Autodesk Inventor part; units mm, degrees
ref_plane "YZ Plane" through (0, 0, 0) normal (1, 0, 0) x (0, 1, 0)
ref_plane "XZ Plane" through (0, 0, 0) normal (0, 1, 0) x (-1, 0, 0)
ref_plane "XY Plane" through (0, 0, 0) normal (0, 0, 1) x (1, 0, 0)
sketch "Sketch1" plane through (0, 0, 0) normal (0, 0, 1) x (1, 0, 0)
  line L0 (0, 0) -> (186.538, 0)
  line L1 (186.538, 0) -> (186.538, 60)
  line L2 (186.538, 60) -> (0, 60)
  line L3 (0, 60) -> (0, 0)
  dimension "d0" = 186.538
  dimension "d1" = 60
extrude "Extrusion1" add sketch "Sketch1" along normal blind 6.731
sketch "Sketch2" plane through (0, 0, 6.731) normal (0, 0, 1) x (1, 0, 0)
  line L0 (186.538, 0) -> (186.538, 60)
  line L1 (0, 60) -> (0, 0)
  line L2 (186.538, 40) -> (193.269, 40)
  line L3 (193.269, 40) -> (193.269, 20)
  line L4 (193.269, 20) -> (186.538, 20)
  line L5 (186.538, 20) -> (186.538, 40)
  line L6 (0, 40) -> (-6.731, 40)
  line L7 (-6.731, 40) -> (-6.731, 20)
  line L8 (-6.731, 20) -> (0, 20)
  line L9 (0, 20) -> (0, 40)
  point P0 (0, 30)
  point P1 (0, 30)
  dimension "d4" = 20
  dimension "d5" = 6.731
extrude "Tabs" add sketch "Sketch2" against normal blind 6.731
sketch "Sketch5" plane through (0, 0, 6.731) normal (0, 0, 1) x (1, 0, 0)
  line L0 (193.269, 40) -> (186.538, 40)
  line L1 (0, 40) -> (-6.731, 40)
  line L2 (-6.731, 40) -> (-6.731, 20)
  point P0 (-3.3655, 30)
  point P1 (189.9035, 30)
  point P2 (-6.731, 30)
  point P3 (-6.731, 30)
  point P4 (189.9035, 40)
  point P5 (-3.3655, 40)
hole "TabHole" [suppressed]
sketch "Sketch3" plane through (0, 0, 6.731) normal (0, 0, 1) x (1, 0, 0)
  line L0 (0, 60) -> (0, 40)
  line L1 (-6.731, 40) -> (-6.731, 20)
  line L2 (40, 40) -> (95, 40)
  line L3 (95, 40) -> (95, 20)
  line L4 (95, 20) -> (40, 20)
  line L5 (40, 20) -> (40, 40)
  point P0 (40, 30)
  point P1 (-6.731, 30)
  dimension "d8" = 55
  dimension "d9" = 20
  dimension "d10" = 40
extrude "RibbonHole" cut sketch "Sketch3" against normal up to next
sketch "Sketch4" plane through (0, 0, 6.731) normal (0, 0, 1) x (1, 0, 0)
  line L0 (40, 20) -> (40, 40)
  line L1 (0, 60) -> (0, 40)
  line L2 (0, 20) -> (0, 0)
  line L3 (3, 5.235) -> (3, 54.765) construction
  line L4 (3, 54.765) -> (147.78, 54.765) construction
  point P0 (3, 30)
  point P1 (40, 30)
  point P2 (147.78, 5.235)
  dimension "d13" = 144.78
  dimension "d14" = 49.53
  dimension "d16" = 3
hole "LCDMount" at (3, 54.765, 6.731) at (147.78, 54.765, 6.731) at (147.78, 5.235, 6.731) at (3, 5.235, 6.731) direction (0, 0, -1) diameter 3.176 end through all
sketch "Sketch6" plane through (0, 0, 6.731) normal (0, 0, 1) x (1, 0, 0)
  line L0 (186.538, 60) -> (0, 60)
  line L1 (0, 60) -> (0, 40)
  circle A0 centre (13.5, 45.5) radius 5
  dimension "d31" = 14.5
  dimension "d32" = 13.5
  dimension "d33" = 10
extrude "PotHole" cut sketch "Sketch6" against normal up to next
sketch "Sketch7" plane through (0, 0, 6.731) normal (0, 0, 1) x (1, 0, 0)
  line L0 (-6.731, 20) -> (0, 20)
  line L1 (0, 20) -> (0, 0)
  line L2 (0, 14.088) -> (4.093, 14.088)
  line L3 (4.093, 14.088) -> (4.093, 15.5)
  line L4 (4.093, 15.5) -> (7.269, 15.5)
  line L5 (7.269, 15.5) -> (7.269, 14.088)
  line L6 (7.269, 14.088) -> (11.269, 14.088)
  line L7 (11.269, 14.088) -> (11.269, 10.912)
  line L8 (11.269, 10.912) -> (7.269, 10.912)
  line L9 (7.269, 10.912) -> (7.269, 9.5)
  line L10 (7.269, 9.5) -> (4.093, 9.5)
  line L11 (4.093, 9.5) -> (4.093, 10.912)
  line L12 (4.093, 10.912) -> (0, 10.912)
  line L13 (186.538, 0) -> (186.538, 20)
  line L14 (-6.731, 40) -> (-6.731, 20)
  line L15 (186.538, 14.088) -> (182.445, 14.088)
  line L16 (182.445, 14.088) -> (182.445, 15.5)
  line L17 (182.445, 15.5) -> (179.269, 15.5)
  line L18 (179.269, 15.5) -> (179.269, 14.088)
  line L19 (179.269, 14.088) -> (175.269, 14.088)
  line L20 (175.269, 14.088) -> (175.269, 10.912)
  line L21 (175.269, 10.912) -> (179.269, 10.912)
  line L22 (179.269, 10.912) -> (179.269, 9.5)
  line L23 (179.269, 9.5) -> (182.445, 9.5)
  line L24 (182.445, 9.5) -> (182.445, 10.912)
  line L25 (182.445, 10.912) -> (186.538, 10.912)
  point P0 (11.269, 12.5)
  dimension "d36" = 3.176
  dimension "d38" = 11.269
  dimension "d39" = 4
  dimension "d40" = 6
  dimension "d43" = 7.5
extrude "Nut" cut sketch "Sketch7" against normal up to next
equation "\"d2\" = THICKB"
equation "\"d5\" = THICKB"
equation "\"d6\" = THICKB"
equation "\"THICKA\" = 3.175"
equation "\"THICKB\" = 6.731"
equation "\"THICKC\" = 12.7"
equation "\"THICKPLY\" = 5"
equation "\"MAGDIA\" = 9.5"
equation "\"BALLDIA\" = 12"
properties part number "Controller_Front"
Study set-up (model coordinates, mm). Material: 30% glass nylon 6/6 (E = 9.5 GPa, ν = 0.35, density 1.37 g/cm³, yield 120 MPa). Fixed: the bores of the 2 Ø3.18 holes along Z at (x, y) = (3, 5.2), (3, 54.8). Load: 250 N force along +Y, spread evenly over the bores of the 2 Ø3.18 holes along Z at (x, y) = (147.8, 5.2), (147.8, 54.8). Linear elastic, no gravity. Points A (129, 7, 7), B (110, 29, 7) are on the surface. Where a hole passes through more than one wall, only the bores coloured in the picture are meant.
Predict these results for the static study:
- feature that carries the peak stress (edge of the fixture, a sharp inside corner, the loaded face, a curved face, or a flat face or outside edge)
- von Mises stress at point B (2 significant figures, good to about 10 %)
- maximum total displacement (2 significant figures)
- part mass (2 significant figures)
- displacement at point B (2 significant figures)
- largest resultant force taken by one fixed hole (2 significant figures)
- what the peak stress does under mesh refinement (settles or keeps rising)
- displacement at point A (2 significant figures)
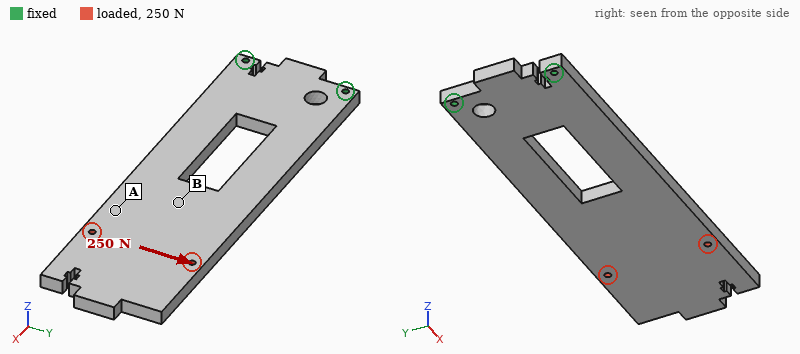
edge of the fixture
3.5 MPa
0.50 mm
94 g
0.28 mm
730 N
keeps rising
0.33 mm
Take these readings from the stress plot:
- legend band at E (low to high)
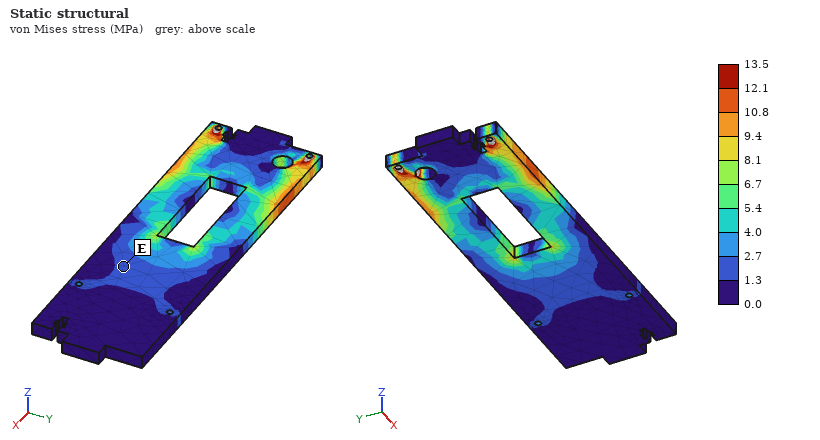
1.3 to 2.7 MPa
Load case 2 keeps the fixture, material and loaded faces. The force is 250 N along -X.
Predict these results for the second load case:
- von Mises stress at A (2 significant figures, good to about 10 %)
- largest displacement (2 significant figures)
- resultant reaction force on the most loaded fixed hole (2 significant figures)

0.79 MPa
16 µm
130 N
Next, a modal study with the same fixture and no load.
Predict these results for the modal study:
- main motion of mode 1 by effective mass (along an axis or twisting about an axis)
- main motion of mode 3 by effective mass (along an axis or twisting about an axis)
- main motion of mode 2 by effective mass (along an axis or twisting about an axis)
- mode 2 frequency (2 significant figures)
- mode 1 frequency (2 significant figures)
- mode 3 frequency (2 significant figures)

along Z
along Z
twisting about X
440 Hz
66 Hz
470 Hz
